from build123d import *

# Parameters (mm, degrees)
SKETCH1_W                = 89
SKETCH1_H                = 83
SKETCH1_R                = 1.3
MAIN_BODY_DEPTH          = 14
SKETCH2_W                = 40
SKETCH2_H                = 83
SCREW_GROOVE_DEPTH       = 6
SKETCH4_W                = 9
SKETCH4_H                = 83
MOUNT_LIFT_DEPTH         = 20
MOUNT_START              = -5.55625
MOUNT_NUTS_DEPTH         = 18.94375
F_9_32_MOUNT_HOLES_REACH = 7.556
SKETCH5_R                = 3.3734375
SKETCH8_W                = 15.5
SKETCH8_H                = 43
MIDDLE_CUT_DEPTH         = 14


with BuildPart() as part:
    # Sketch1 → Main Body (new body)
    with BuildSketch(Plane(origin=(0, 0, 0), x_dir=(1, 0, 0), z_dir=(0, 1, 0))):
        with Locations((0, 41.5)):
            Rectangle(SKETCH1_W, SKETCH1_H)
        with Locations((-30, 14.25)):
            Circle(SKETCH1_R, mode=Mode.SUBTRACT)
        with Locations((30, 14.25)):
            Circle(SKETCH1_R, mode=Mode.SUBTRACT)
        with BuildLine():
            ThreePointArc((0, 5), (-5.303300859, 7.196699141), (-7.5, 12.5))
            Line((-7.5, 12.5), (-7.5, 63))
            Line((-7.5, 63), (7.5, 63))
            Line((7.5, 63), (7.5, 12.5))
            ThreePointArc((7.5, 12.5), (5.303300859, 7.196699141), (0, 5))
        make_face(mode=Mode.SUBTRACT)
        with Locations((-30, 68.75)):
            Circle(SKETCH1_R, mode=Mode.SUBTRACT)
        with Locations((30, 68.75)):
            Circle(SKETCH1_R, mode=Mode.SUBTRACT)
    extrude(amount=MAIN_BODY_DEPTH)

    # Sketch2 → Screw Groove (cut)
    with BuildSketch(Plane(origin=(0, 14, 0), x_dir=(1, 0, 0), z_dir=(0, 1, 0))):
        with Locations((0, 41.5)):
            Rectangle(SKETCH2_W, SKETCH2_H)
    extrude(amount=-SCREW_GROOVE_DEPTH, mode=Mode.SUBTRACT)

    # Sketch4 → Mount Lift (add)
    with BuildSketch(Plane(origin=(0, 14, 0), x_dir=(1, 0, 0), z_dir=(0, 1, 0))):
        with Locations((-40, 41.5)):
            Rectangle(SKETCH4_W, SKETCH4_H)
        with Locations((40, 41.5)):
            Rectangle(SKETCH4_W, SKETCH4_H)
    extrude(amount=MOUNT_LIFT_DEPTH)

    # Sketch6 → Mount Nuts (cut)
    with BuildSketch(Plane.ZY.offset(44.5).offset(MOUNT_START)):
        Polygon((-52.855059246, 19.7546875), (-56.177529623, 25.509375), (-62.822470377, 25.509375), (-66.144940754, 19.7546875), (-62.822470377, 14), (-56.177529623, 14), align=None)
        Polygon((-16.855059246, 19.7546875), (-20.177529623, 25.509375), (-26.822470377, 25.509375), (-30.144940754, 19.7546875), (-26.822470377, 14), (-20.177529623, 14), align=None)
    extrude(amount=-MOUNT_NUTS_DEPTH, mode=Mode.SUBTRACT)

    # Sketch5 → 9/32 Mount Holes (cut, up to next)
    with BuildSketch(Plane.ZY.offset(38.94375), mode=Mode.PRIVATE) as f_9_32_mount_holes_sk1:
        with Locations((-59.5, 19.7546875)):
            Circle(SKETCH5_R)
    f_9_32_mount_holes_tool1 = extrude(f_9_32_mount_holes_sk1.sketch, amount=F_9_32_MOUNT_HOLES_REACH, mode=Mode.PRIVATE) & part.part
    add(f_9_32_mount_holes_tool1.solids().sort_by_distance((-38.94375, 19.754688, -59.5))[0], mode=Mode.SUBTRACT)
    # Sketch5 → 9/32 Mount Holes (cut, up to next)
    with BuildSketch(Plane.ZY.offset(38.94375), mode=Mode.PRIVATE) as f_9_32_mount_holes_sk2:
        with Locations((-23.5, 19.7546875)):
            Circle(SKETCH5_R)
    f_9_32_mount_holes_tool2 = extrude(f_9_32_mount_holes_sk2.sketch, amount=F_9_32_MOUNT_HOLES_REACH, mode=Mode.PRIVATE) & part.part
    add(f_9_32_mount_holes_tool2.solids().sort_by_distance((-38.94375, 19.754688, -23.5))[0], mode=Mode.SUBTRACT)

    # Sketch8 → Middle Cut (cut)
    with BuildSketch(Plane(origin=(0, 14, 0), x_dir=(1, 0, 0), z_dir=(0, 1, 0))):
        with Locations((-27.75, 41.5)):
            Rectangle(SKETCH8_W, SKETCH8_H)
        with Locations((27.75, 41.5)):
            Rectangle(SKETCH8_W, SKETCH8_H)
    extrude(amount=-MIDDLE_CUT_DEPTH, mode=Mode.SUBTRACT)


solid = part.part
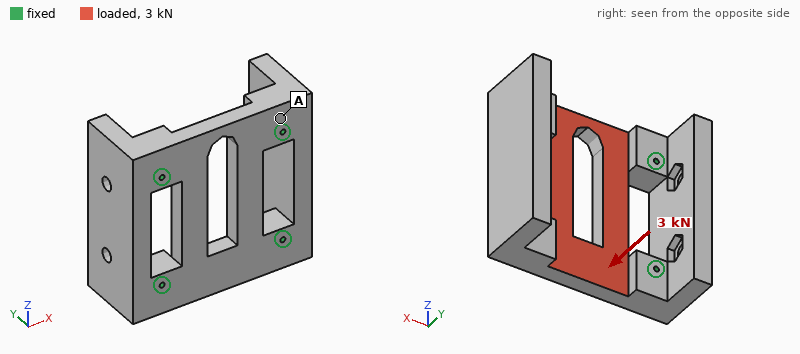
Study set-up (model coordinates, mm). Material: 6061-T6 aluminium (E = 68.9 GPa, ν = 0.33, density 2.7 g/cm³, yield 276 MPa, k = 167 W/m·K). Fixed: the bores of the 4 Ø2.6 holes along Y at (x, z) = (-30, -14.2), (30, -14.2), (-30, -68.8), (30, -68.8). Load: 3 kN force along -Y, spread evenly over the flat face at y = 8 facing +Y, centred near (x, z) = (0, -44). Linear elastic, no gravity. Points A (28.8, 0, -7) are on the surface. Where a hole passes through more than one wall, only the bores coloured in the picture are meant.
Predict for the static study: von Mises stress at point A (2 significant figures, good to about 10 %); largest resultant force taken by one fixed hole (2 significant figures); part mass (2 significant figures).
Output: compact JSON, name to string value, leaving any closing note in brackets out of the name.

{"von Mises stress at point A": "7.3 MPa", "largest resultant force taken by one fixed hole": "880 N", "part mass": "230 g"}
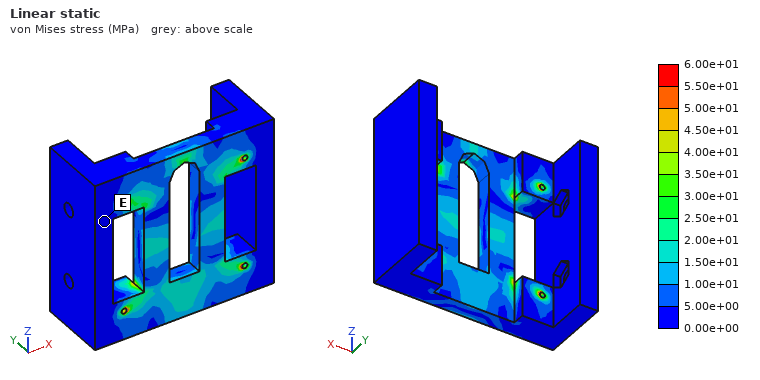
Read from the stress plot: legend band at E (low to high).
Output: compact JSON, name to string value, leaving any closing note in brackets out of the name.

{"legend band at E": "0.00e+00 to 5.00e+00 MPa"}
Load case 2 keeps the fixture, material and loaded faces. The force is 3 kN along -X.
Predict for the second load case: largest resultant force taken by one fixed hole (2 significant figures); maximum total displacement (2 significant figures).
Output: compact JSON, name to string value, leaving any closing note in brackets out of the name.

{"largest resultant force taken by one fixed hole": "860 N", "maximum total displacement": "9.8 µm"}
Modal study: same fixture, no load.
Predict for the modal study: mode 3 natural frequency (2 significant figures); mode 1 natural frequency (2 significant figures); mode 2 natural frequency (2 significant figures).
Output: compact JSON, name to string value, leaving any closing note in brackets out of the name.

{"mode 3 natural frequency": "8800 Hz", "mode 1 natural frequency": "6100 Hz", "mode 2 natural frequency": "6200 Hz"}
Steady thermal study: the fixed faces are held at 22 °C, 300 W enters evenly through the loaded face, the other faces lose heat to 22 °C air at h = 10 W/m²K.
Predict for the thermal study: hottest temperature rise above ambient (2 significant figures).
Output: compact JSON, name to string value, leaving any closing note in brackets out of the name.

{"hottest temperature rise above ambient": "66 K"}
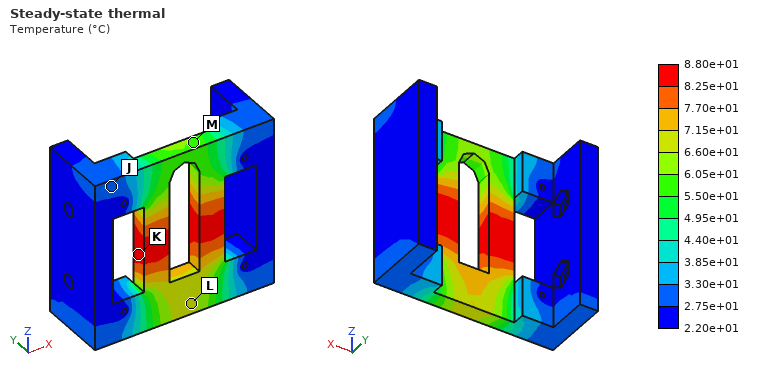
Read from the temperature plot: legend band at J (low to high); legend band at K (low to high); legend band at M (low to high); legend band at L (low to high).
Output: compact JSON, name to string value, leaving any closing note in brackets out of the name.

{"legend band at J": "2.75e+01 to 3.30e+01 °C", "legend band at K": "8.25e+01 to 8.80e+01 °C", "legend band at M": "5.50e+01 to 6.05e+01 °C", "legend band at L": "6.60e+01 to 7.15e+01 °C"}
